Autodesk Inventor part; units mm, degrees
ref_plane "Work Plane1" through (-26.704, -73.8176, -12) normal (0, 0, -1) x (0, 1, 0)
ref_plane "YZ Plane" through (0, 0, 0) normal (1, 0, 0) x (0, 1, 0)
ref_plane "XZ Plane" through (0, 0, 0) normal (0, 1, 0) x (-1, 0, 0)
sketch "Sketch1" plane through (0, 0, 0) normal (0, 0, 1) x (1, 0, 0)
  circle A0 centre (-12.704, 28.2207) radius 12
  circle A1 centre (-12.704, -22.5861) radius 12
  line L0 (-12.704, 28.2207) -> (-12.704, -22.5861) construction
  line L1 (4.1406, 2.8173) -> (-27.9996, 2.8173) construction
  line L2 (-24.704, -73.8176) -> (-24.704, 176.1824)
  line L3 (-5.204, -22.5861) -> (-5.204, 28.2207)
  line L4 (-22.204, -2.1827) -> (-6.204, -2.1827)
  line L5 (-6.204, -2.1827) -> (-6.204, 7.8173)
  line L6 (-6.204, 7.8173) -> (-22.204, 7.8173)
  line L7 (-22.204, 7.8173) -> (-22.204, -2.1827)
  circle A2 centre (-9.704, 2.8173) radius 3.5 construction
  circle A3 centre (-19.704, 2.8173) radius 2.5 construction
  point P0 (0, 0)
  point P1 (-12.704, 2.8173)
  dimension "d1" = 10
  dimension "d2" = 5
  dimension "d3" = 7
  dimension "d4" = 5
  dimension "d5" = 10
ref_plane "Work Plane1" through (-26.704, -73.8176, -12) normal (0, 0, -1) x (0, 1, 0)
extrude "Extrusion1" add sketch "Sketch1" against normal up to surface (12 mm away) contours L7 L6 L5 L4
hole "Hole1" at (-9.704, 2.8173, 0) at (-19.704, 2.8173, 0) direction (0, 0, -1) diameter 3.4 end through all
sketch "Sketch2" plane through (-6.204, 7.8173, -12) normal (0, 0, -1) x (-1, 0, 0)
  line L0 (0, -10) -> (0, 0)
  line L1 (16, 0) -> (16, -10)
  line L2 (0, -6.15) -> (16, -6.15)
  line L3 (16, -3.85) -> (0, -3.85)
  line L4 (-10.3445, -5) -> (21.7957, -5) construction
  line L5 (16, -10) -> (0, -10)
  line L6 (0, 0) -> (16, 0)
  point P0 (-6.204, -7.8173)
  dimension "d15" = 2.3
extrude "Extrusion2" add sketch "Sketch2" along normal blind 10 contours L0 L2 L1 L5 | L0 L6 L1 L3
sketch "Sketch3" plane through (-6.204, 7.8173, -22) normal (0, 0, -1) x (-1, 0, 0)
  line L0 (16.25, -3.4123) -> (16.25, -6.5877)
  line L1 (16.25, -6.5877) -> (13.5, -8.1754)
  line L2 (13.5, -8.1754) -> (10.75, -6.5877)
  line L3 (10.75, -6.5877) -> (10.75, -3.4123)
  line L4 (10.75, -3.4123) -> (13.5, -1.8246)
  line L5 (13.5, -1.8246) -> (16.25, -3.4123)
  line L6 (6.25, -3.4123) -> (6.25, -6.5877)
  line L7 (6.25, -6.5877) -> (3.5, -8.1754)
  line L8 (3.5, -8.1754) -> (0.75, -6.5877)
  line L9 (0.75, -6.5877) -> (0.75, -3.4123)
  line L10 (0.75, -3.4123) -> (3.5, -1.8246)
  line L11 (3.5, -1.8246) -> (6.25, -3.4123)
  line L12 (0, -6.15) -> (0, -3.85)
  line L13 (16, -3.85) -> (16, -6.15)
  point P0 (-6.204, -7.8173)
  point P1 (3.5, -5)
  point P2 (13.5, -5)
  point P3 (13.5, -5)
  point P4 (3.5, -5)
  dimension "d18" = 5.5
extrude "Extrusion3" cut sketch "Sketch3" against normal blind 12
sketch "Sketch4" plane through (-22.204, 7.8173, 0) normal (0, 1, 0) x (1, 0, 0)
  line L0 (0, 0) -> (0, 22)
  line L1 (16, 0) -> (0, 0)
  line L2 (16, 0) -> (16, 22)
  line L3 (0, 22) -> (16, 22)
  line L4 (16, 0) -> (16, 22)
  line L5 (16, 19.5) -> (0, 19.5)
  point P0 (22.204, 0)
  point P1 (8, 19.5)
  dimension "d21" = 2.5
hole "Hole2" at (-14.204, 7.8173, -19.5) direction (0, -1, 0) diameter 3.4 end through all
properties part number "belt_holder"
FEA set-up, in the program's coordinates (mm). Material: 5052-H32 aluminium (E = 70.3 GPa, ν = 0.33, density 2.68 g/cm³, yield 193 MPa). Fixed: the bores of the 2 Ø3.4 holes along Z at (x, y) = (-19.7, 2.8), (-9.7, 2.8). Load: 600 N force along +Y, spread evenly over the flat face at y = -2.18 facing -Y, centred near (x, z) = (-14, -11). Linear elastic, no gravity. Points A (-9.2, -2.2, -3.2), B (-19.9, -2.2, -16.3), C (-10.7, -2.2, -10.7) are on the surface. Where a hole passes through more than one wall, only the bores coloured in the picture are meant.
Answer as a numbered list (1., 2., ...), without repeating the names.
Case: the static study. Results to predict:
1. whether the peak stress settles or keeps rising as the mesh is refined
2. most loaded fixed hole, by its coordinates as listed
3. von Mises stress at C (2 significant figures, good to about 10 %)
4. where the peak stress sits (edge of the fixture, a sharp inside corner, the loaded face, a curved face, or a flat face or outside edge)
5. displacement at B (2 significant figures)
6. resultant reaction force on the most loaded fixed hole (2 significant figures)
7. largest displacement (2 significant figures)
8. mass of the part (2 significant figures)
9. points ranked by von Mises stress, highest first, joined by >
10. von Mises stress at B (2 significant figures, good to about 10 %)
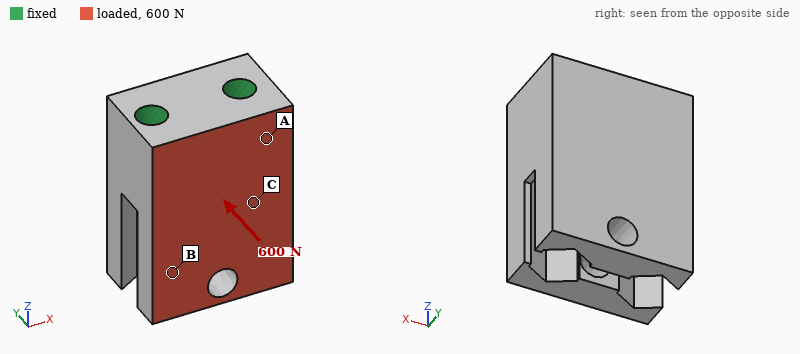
1. keeps rising
2. (-9.7, 2.8)
3. 36 MPa
4. a sharp inside corner
5. 13 µm
6. 320 N
7. 28 µm
8. 6.8 g
9. C > B > A
10. 13 MPa
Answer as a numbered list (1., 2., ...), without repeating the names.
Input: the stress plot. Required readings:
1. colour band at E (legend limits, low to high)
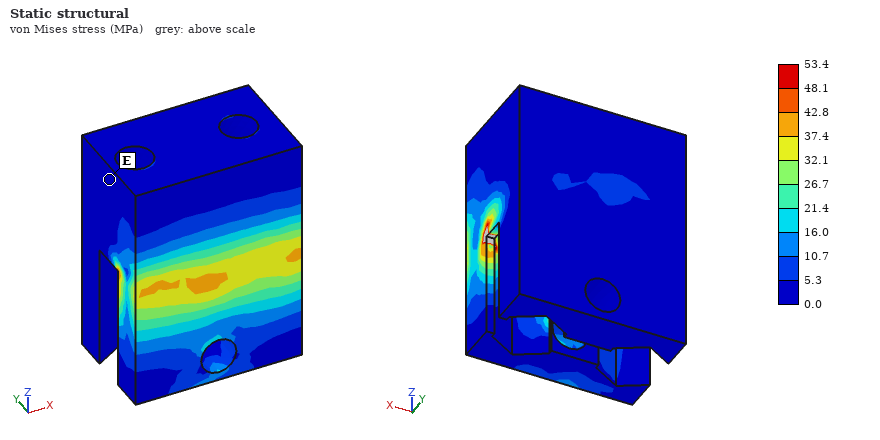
1. 0.0 to 5.3 MPa
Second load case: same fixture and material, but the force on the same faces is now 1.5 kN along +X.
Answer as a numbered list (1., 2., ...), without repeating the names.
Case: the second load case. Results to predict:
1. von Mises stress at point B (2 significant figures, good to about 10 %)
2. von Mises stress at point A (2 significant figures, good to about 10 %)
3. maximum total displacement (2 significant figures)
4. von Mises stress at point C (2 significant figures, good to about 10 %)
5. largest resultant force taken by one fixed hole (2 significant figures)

1. 33 MPa
2. 10 MPa
3. 22 µm
4. 32 MPa
5. 1.1 kN
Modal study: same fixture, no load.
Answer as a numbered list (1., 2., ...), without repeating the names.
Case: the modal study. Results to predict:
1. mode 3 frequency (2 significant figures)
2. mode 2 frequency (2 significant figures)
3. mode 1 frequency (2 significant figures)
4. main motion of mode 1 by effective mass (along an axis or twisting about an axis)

1. 27 kHz
2. 19 kHz
3. 18 kHz
4. along Y
